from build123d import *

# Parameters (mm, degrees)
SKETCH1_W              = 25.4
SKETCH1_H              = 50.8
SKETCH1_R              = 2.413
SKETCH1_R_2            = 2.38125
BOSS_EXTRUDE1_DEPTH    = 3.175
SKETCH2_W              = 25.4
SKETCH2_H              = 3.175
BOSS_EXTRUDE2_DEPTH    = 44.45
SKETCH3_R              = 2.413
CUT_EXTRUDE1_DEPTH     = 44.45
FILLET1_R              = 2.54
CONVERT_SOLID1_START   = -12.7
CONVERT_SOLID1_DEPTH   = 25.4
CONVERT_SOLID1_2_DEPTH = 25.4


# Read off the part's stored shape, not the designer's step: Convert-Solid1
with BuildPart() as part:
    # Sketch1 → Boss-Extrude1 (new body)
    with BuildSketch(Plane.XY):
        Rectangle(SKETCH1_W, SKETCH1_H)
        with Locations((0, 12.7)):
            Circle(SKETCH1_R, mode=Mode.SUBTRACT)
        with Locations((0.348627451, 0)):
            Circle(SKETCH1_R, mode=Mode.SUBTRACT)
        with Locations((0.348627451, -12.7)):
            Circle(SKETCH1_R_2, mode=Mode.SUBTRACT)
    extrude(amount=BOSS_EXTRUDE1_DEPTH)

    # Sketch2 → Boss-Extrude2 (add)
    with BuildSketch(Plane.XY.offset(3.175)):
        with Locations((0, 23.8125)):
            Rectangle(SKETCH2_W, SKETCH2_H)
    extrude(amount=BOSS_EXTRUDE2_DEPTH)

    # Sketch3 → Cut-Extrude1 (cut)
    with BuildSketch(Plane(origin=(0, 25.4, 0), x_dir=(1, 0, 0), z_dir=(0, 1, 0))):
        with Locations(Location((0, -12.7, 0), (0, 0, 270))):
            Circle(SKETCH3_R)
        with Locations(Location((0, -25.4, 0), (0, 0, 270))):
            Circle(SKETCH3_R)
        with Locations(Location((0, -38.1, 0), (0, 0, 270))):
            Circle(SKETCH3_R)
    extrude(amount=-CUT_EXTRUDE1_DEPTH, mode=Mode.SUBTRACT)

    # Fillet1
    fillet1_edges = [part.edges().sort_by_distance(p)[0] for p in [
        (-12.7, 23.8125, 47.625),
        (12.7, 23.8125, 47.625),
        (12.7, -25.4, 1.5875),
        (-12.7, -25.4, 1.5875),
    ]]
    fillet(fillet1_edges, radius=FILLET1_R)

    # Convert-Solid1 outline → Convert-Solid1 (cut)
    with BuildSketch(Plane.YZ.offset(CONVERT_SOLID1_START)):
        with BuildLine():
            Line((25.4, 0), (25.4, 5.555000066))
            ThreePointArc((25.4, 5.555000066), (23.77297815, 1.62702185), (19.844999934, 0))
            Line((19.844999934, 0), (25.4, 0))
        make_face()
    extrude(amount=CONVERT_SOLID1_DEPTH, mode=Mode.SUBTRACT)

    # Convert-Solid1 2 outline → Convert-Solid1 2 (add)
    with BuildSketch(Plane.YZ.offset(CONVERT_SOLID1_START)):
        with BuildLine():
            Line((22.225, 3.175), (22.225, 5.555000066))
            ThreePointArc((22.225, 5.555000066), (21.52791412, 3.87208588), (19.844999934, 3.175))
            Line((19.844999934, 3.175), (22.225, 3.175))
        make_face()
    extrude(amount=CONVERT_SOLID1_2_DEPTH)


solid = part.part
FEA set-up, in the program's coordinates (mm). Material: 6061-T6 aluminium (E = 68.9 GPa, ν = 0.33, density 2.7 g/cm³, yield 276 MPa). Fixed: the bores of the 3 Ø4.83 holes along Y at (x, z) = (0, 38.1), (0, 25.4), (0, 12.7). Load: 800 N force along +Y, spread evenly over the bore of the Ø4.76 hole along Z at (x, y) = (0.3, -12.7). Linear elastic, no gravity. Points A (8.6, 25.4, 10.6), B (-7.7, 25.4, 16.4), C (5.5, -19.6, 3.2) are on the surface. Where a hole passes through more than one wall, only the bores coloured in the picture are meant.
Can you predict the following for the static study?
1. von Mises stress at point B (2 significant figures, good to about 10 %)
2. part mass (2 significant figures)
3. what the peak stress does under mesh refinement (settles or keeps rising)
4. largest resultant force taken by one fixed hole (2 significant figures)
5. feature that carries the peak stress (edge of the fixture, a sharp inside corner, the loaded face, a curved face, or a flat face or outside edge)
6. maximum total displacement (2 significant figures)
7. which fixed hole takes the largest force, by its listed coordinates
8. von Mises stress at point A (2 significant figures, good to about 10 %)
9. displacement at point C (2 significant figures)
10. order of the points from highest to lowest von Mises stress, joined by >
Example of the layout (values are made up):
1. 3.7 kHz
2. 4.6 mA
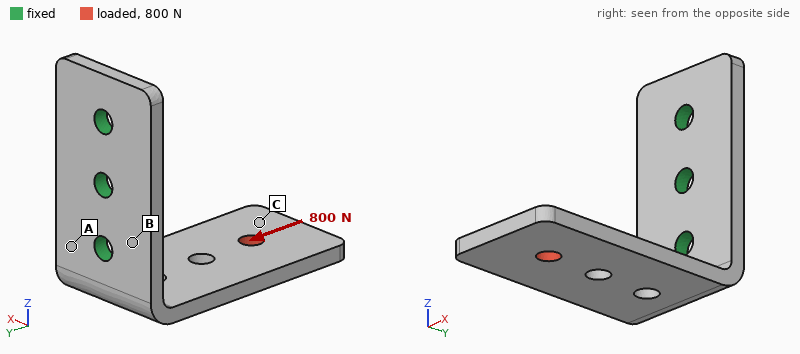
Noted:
1. 35 MPa
2. 19 g
3. keeps rising
4. 970 N
5. edge of the fixture
6. 0.50 mm
7. (0, 12.7)
8. 85 MPa
9. 0.43 mm
10. A > B > C
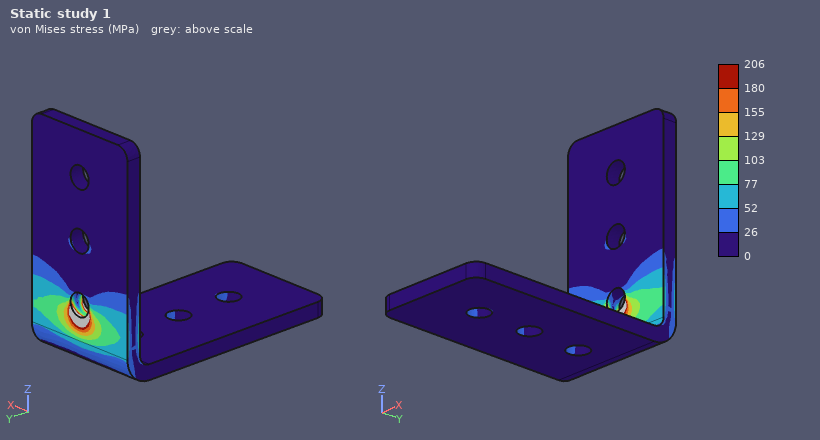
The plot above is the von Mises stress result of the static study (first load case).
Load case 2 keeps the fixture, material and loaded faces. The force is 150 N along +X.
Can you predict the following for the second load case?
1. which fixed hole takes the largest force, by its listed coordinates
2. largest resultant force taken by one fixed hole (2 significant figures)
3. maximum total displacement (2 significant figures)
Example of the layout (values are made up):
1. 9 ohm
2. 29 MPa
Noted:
1. (0, 12.7)
2. 200 N
3. 0.34 mm
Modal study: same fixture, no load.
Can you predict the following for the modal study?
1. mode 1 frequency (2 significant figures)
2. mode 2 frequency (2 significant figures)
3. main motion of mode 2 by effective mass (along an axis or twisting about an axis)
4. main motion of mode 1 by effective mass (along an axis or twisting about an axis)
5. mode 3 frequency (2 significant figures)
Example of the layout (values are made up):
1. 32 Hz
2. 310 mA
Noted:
1. 820 Hz
2. 1500 Hz
3. along X
4. along Z
5. 4000 Hz
